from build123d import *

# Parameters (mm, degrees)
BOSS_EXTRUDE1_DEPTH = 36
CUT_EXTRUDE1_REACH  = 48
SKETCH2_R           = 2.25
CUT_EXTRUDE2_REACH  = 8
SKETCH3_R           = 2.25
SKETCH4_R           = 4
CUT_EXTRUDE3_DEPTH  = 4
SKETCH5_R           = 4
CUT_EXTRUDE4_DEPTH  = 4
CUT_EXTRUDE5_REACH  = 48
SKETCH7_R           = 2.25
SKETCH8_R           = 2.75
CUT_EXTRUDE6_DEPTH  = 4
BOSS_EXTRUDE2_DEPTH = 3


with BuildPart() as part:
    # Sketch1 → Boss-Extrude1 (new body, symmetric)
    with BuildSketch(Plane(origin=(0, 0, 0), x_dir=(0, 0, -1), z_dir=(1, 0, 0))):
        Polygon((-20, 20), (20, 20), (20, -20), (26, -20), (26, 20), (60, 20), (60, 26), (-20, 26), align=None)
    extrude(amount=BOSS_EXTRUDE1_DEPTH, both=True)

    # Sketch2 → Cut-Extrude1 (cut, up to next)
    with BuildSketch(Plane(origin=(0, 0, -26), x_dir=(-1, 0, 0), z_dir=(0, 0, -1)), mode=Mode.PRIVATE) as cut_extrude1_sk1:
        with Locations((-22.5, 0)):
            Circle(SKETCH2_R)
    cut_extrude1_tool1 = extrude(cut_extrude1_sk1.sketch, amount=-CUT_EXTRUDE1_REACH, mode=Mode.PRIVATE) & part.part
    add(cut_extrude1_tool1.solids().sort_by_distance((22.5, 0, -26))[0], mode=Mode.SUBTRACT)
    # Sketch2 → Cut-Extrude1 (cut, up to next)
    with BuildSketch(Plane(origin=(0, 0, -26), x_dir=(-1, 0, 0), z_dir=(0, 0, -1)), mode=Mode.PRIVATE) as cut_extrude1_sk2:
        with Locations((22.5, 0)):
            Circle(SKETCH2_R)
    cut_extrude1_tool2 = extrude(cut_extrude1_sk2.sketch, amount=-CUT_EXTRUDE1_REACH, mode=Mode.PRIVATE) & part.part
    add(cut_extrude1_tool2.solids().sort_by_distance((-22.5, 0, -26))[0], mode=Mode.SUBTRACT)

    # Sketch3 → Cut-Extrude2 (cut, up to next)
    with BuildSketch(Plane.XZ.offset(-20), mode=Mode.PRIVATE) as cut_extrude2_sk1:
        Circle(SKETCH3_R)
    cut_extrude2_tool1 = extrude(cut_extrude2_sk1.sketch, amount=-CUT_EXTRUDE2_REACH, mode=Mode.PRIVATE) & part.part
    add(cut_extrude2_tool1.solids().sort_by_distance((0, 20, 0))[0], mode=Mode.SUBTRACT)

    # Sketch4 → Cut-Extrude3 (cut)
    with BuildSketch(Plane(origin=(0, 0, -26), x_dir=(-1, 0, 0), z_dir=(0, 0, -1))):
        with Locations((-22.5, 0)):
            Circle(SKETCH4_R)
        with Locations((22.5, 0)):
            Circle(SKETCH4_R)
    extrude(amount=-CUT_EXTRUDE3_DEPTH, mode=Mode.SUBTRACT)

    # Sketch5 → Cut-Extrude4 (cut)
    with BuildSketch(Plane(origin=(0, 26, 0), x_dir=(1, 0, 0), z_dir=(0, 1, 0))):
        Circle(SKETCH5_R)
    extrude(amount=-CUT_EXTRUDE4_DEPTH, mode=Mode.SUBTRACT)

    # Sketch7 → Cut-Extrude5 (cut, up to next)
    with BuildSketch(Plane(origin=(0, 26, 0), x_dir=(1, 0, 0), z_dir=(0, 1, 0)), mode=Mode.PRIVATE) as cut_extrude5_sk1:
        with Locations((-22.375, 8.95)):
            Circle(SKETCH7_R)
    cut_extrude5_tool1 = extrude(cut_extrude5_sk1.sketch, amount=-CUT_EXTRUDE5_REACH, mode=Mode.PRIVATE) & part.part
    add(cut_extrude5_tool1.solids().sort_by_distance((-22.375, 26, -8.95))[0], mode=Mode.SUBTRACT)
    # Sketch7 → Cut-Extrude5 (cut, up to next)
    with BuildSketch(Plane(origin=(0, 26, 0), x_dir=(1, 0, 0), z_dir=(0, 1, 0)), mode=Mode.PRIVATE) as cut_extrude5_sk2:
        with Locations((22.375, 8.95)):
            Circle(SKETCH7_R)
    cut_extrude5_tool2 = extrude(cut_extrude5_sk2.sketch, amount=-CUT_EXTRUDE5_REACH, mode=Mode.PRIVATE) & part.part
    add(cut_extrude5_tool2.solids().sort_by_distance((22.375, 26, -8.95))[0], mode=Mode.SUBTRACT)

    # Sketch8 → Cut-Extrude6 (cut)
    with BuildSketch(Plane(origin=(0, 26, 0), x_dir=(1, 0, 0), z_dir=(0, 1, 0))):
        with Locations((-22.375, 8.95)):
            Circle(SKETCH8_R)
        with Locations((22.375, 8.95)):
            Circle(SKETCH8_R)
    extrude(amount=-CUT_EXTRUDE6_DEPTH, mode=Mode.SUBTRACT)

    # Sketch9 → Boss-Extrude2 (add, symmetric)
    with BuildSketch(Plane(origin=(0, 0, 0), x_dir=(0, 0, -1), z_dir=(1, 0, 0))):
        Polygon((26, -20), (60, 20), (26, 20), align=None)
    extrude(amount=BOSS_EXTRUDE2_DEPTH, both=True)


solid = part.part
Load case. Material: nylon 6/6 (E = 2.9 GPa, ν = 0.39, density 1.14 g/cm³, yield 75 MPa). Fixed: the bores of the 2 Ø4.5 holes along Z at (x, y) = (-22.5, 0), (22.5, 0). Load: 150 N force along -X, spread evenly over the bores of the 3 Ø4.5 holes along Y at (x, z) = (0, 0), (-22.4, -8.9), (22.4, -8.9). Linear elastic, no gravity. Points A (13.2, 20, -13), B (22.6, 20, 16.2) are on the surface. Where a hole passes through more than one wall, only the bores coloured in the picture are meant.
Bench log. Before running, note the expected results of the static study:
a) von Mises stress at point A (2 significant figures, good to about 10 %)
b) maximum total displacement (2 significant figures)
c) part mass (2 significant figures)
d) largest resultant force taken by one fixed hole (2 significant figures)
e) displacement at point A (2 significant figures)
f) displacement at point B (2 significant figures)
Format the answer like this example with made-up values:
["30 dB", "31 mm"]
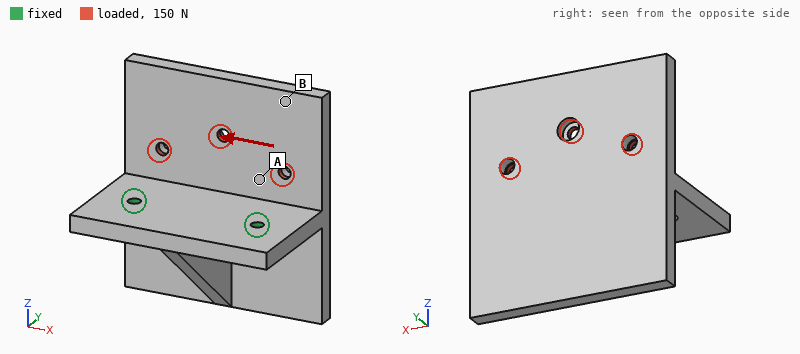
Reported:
["1.6 MPa", "0.24 mm", "63 g", "110 N", "0.077 mm", "0.20 mm"]
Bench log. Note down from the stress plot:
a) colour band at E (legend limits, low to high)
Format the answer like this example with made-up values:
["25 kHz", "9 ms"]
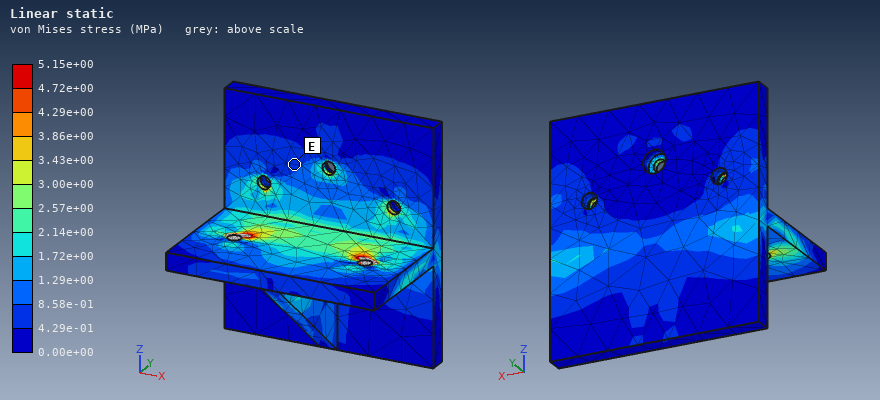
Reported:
["4.29e-01 to 8.58e-01 MPa"]
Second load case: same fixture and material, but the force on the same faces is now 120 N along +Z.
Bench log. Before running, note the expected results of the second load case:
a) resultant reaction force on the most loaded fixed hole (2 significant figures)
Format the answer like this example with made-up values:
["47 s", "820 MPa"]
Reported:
["61 N"]
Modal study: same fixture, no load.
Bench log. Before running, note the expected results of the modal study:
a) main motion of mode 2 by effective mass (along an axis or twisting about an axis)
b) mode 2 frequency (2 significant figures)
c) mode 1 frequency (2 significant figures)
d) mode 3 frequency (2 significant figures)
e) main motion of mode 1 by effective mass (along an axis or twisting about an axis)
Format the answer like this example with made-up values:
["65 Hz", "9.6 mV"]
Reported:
["twisting about Y", "680 Hz", "230 Hz", "900 Hz", "along Z"]
